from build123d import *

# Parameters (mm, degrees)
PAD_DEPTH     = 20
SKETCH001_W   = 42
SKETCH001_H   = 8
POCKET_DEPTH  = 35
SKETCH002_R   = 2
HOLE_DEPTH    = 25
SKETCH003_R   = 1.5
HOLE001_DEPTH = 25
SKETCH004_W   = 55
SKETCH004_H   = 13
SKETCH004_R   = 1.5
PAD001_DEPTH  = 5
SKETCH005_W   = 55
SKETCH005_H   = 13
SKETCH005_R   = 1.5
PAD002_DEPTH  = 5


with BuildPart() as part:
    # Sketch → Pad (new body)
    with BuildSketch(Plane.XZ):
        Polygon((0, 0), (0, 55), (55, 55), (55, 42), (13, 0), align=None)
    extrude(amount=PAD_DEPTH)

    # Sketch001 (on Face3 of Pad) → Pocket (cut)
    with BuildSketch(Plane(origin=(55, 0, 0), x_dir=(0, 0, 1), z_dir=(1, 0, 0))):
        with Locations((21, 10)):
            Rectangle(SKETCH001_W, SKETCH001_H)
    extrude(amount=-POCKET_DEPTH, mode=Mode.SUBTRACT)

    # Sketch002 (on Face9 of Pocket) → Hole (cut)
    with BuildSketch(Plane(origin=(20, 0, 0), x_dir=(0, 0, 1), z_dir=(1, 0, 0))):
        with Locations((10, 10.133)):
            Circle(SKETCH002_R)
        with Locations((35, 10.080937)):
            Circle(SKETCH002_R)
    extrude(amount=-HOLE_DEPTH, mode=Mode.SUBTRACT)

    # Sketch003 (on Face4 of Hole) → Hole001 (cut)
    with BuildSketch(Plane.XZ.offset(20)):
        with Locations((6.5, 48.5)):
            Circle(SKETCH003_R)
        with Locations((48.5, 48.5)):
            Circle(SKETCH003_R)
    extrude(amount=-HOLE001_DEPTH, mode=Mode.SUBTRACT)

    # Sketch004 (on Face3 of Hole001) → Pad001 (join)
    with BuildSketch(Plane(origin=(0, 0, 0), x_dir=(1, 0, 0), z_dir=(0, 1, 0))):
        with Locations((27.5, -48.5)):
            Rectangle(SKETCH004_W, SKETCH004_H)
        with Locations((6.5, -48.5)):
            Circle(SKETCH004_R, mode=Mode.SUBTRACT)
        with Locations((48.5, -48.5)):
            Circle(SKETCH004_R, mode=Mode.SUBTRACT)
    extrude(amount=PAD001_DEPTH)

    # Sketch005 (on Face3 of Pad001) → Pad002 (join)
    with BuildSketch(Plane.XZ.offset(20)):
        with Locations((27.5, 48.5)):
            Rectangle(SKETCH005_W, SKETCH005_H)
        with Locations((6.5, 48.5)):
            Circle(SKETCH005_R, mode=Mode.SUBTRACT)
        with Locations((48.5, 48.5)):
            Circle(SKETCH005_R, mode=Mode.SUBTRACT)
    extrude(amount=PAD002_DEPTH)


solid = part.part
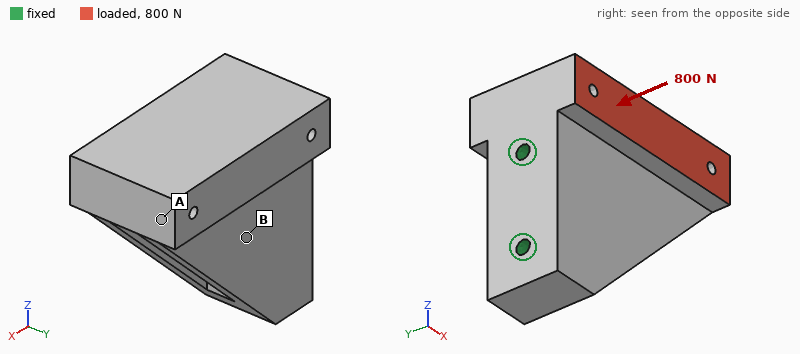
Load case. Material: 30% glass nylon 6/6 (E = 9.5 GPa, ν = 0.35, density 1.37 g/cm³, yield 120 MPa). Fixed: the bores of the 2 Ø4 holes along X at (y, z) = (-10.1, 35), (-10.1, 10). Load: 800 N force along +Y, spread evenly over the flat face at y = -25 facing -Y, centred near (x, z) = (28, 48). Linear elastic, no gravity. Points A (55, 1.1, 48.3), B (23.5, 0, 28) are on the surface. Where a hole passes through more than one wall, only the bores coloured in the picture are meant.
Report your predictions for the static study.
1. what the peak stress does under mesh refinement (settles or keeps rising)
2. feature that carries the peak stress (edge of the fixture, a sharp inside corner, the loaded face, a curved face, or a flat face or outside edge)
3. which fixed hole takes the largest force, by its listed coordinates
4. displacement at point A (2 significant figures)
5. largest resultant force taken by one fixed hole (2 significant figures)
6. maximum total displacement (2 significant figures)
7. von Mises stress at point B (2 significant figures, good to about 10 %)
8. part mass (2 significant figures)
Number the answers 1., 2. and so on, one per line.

1. keeps rising
2. edge of the fixture
3. (-10.1, 35)
4. 88 µm
5. 1.1 kN
6. 96 µm
7. 6.1 MPa
8. 61 g
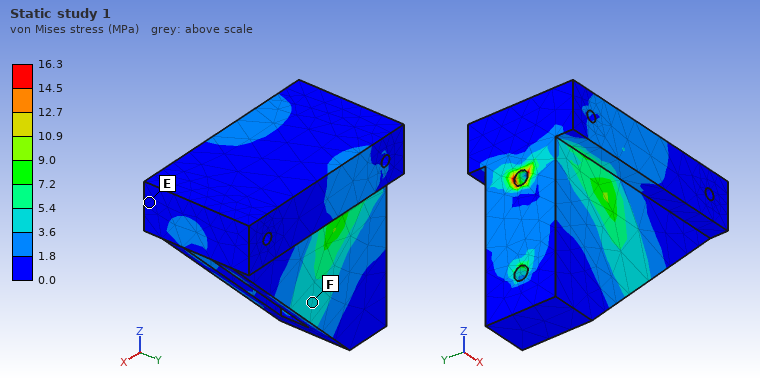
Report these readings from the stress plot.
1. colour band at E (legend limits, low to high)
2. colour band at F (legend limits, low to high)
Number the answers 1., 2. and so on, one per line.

1. 0.0 to 1.8 MPa
2. 3.6 to 5.4 MPa
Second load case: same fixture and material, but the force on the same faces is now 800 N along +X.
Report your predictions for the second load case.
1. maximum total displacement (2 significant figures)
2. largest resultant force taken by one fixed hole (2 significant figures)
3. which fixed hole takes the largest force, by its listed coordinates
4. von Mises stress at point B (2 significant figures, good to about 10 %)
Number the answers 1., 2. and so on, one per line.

1. 82 µm
2. 950 N
3. (-10.1, 35)
4. 4.1 MPa
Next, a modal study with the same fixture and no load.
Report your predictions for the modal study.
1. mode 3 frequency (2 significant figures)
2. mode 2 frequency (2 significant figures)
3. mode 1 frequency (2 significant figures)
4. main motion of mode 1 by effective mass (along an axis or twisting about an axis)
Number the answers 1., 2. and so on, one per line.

1. 5800 Hz
2. 4800 Hz
3. 3000 Hz
4. along Y
